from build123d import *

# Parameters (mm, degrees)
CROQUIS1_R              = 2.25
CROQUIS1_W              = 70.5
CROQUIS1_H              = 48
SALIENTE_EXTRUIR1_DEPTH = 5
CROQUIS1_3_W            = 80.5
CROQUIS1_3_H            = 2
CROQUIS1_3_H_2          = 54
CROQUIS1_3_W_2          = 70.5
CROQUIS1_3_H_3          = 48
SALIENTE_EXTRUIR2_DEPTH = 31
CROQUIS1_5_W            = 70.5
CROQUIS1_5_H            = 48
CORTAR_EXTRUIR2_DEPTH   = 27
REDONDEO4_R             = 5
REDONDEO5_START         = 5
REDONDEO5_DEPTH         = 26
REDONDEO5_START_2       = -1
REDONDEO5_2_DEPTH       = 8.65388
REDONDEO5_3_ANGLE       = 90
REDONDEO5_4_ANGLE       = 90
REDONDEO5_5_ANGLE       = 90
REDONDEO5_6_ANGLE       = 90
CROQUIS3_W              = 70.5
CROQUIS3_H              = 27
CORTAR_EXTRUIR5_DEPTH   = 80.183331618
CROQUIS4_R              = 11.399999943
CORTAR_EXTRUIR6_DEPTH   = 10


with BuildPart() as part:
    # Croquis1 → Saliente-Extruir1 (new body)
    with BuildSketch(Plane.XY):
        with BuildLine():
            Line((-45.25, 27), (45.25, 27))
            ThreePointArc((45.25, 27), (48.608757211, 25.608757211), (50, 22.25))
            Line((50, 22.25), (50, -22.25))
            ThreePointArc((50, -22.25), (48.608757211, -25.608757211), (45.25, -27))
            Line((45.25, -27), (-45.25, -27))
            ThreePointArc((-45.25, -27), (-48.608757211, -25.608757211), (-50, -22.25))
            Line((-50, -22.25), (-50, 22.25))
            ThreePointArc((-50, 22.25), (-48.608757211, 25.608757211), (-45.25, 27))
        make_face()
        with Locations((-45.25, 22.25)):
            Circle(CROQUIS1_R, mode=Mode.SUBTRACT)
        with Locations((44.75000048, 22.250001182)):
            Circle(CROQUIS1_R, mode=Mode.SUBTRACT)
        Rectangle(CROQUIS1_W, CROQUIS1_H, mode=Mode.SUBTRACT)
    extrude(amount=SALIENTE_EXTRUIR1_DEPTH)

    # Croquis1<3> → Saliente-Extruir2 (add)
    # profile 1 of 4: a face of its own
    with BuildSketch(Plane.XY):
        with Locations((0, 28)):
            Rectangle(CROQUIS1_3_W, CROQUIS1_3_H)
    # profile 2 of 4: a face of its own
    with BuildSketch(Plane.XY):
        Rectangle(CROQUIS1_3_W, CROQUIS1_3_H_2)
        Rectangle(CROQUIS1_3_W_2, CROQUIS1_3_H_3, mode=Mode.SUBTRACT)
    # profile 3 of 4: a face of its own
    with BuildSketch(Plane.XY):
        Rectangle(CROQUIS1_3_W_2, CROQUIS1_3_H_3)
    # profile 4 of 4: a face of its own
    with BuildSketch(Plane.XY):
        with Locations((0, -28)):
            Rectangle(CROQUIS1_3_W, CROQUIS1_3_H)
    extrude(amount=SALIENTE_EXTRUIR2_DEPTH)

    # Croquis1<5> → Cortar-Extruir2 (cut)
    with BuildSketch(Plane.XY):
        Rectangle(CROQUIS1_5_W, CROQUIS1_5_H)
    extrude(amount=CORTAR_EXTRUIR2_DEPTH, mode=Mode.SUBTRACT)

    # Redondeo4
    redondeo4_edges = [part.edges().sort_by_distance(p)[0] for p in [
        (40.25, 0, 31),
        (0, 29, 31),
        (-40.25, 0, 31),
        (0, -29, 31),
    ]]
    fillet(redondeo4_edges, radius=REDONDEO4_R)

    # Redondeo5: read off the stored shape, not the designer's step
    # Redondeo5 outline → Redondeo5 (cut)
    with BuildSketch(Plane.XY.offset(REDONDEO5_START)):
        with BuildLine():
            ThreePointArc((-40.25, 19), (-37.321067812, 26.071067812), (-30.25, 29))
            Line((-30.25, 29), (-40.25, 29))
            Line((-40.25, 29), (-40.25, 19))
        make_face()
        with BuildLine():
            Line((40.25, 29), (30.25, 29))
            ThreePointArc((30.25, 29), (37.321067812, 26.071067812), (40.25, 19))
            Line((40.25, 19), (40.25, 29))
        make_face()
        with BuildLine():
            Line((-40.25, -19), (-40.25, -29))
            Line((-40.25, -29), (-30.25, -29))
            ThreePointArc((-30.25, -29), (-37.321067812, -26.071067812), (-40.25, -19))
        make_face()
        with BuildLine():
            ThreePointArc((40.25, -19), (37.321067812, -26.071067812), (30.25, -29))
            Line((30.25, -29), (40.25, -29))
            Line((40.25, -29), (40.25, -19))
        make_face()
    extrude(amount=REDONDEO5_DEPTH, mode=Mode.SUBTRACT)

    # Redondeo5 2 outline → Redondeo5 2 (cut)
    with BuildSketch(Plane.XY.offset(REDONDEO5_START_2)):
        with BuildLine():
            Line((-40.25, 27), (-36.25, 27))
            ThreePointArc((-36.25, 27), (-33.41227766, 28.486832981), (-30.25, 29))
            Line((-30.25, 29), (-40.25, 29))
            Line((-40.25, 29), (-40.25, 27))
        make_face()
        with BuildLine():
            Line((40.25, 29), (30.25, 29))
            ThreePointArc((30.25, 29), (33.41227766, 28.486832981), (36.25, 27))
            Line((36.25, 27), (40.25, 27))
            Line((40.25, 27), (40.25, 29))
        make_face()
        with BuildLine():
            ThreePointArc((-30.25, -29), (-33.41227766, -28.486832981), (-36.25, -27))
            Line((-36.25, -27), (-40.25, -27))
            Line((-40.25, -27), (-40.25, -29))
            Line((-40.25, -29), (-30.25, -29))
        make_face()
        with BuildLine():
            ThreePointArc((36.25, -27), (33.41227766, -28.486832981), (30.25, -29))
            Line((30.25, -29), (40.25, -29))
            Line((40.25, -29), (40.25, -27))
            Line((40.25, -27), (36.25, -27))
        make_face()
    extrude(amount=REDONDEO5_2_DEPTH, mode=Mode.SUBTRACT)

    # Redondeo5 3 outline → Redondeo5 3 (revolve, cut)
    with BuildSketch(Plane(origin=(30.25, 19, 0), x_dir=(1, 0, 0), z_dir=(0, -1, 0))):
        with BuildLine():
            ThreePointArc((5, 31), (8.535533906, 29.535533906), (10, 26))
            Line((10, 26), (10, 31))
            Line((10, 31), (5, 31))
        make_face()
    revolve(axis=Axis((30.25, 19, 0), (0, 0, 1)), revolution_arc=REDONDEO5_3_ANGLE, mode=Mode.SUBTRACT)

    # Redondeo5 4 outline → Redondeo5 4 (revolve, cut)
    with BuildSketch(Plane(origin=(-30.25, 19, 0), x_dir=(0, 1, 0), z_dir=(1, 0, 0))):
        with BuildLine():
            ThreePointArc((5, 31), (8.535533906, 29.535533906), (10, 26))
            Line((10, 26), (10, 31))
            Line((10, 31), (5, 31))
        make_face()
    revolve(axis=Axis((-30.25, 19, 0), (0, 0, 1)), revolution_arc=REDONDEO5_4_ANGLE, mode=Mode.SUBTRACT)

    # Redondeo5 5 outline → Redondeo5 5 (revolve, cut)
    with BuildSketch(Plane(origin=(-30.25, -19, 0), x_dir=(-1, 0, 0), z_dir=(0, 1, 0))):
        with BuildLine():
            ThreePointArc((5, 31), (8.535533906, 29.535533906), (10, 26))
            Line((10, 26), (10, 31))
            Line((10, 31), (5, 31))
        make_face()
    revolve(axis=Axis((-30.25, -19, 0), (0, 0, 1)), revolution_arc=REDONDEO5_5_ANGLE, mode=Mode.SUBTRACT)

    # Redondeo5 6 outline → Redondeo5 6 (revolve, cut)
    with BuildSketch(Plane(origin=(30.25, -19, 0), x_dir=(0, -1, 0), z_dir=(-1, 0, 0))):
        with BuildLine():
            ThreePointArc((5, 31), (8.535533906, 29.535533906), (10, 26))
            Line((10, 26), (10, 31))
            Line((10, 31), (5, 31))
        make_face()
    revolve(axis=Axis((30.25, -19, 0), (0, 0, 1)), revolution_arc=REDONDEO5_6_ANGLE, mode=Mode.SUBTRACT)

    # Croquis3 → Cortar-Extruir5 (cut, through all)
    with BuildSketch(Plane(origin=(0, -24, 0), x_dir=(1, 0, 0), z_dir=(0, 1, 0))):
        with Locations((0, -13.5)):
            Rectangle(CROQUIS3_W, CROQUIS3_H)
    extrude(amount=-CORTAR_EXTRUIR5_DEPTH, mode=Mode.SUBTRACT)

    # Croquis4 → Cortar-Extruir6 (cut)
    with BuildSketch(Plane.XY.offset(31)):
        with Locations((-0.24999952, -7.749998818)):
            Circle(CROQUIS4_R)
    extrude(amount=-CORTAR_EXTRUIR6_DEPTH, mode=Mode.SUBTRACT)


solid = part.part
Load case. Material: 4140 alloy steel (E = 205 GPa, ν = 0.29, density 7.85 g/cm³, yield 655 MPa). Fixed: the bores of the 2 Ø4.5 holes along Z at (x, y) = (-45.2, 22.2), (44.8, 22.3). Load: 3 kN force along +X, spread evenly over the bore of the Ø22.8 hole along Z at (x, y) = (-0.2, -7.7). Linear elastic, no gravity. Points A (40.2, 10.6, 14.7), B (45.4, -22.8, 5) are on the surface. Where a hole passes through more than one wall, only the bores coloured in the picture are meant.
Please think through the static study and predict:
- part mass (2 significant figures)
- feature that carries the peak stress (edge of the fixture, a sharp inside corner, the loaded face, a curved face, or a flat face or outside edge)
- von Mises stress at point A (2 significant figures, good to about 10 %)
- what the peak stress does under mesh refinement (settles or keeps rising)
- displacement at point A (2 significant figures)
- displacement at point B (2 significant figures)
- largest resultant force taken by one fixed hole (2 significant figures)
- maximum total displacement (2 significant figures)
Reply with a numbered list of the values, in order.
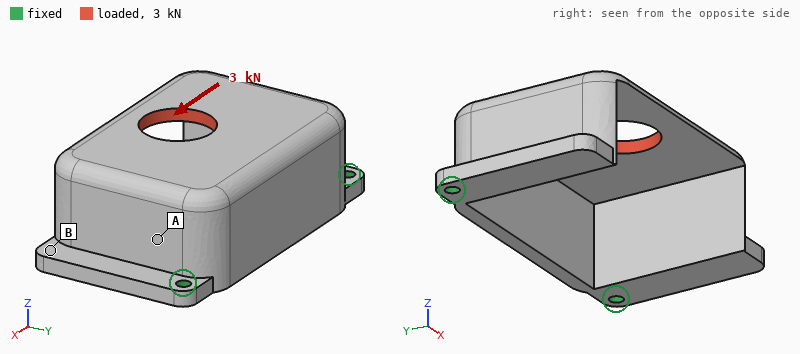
1. 340 g
2. edge of the fixture
3. 33 MPa
4. keeps rising
5. 0.035 mm
6. 0.082 mm
7. 2.0 kN
8. 0.15 mm
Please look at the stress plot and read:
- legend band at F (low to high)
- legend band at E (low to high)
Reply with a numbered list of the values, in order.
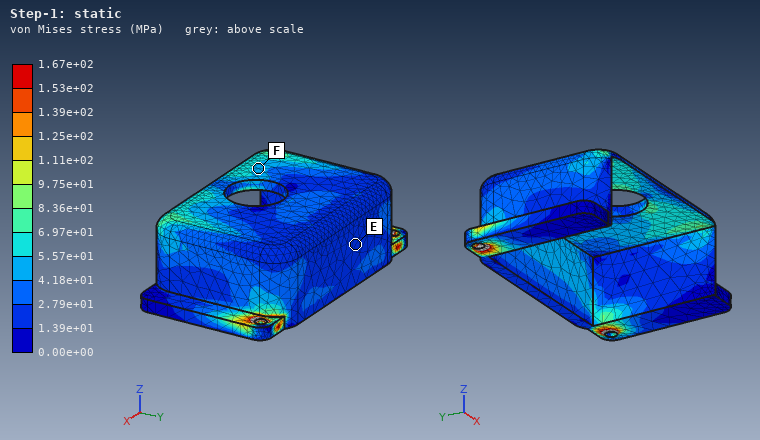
1. 4.18e+01 to 5.57e+01 MPa
2. 1.39e+01 to 2.79e+01 MPa
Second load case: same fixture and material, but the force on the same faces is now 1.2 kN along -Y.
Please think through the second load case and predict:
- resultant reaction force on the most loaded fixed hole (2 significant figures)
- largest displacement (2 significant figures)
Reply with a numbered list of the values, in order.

1. 620 N
2. 0.13 mm
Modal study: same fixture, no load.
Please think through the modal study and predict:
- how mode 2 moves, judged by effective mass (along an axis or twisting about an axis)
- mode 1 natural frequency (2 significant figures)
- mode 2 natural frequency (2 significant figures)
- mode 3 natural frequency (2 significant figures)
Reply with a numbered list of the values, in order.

1. along X
2. 1100 Hz
3. 1700 Hz
4. 3700 Hz
